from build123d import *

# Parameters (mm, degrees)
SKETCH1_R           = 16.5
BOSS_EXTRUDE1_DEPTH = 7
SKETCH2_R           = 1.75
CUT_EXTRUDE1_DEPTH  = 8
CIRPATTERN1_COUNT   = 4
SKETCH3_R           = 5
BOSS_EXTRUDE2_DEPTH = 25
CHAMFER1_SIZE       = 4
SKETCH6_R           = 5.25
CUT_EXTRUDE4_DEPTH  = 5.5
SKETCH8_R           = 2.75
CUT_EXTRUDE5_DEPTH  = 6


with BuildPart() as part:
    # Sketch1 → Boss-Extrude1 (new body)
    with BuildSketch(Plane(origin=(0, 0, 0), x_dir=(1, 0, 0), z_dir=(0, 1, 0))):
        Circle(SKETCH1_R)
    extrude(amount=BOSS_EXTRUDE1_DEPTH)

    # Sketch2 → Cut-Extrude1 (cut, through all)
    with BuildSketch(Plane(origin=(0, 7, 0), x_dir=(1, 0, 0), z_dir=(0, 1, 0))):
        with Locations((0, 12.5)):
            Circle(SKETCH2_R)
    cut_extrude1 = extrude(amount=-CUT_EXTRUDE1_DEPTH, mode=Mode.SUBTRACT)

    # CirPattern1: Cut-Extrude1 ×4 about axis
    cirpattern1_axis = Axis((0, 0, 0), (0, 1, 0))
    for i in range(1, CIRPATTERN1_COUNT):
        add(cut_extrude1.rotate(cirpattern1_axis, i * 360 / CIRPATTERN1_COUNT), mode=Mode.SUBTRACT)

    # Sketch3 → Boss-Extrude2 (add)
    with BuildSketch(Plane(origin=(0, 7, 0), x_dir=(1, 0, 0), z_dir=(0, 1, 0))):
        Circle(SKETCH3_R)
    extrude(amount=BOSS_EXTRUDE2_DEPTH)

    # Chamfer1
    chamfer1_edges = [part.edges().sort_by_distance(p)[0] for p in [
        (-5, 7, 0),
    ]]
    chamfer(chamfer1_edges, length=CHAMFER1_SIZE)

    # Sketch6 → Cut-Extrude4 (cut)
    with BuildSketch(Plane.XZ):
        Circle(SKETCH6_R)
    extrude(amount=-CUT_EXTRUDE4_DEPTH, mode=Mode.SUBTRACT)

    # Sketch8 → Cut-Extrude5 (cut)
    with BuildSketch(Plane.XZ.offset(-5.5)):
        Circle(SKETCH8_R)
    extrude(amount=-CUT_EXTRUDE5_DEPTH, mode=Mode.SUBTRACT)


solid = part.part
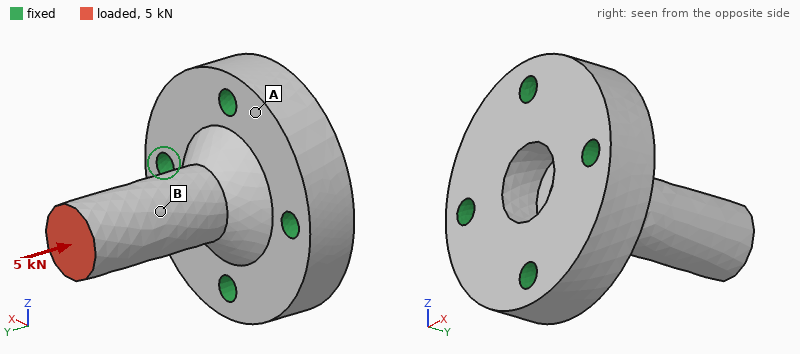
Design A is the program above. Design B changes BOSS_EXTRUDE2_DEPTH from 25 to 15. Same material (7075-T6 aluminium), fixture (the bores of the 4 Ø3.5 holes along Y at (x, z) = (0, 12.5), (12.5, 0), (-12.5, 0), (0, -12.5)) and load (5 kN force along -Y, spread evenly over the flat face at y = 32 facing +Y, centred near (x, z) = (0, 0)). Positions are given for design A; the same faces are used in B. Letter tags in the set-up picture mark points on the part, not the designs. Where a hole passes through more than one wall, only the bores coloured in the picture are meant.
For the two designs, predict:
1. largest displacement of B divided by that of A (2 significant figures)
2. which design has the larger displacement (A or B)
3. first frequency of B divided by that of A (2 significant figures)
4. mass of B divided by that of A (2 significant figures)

0.69
A
2.5
0.89
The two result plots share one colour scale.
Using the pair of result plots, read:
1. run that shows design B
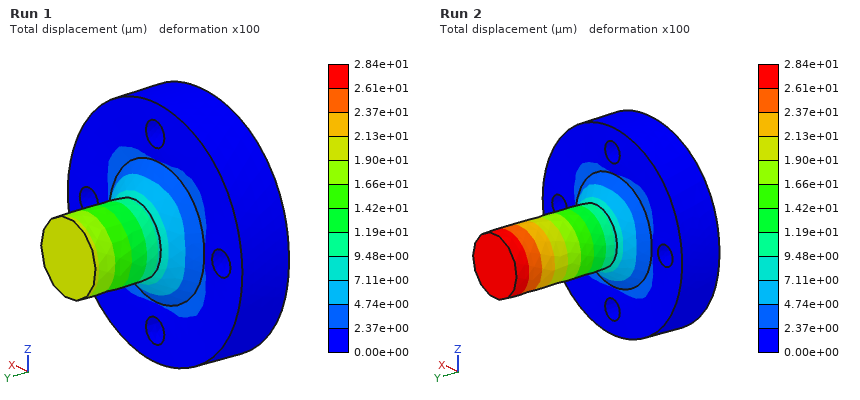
Run 1
